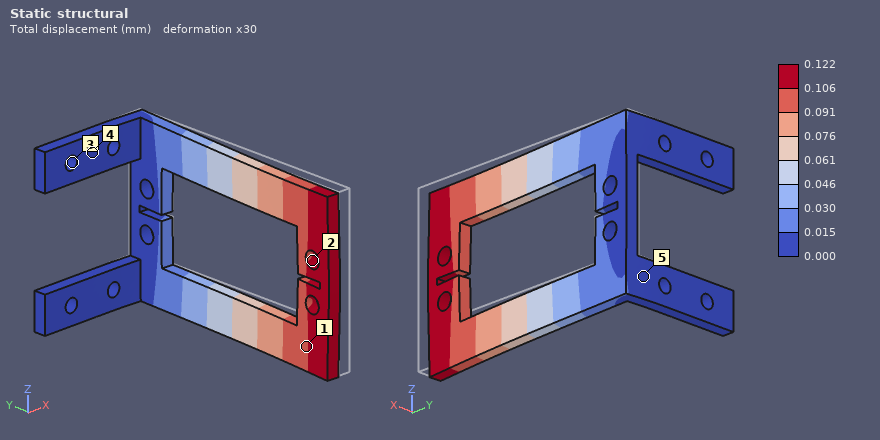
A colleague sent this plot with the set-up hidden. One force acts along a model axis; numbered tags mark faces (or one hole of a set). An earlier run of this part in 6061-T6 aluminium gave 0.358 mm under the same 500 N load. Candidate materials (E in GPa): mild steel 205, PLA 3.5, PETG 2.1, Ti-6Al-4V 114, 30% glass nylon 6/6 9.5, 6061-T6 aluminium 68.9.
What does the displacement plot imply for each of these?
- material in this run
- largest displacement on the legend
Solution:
mild steel
0.122 mm
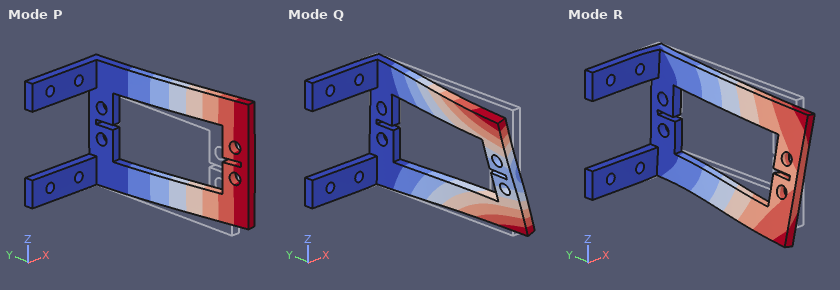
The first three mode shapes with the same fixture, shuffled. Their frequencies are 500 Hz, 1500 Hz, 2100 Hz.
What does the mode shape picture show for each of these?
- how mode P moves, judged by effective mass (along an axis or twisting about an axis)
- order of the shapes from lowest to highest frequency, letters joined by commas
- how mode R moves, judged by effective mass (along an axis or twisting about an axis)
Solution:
along X
P, Q, R
along Z
